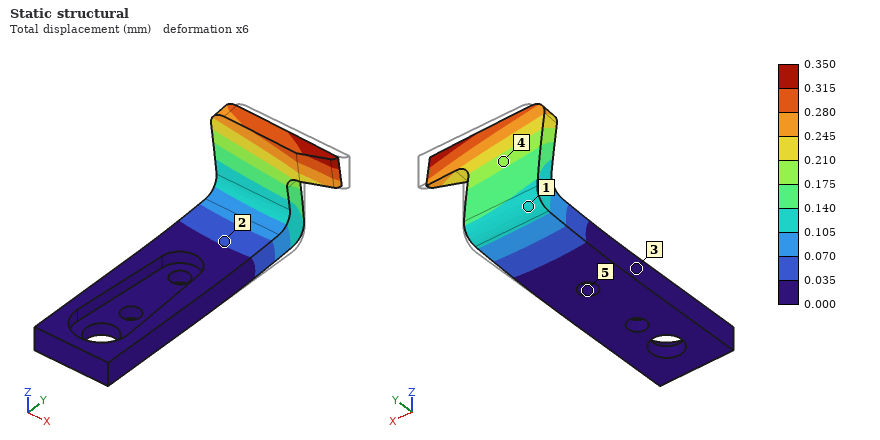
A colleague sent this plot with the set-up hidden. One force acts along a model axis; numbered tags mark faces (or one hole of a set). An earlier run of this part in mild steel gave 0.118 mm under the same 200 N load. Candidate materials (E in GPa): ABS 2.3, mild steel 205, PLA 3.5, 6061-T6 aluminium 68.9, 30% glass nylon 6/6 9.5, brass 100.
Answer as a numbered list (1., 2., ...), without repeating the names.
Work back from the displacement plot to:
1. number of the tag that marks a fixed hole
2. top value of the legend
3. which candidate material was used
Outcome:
1. 5
2. 0.350 mm
3. 6061-T6 aluminium
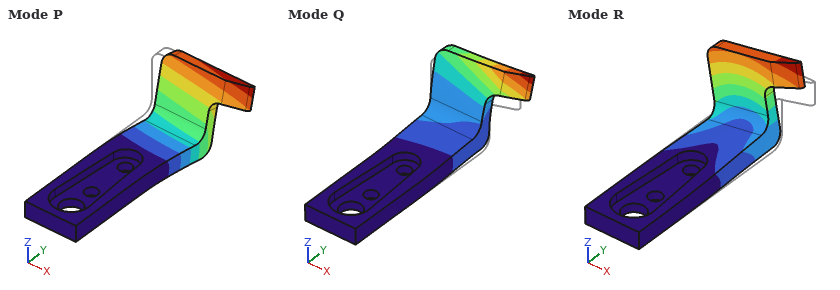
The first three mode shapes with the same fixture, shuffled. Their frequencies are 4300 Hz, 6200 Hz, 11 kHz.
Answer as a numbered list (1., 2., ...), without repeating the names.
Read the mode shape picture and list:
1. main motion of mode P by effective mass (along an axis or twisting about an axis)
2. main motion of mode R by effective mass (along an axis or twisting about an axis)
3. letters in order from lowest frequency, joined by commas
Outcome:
1. along Z
2. along X
3. P, R, Q
